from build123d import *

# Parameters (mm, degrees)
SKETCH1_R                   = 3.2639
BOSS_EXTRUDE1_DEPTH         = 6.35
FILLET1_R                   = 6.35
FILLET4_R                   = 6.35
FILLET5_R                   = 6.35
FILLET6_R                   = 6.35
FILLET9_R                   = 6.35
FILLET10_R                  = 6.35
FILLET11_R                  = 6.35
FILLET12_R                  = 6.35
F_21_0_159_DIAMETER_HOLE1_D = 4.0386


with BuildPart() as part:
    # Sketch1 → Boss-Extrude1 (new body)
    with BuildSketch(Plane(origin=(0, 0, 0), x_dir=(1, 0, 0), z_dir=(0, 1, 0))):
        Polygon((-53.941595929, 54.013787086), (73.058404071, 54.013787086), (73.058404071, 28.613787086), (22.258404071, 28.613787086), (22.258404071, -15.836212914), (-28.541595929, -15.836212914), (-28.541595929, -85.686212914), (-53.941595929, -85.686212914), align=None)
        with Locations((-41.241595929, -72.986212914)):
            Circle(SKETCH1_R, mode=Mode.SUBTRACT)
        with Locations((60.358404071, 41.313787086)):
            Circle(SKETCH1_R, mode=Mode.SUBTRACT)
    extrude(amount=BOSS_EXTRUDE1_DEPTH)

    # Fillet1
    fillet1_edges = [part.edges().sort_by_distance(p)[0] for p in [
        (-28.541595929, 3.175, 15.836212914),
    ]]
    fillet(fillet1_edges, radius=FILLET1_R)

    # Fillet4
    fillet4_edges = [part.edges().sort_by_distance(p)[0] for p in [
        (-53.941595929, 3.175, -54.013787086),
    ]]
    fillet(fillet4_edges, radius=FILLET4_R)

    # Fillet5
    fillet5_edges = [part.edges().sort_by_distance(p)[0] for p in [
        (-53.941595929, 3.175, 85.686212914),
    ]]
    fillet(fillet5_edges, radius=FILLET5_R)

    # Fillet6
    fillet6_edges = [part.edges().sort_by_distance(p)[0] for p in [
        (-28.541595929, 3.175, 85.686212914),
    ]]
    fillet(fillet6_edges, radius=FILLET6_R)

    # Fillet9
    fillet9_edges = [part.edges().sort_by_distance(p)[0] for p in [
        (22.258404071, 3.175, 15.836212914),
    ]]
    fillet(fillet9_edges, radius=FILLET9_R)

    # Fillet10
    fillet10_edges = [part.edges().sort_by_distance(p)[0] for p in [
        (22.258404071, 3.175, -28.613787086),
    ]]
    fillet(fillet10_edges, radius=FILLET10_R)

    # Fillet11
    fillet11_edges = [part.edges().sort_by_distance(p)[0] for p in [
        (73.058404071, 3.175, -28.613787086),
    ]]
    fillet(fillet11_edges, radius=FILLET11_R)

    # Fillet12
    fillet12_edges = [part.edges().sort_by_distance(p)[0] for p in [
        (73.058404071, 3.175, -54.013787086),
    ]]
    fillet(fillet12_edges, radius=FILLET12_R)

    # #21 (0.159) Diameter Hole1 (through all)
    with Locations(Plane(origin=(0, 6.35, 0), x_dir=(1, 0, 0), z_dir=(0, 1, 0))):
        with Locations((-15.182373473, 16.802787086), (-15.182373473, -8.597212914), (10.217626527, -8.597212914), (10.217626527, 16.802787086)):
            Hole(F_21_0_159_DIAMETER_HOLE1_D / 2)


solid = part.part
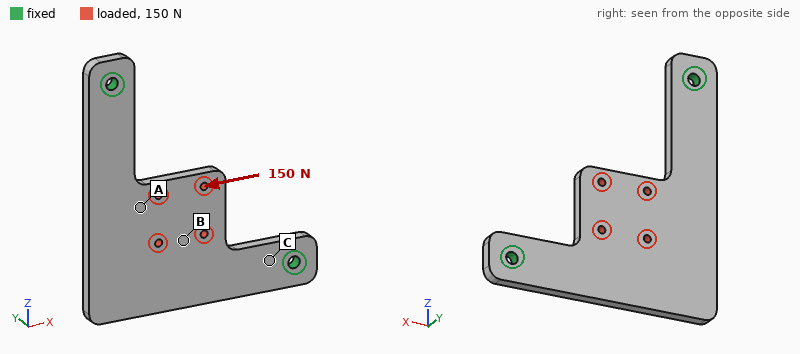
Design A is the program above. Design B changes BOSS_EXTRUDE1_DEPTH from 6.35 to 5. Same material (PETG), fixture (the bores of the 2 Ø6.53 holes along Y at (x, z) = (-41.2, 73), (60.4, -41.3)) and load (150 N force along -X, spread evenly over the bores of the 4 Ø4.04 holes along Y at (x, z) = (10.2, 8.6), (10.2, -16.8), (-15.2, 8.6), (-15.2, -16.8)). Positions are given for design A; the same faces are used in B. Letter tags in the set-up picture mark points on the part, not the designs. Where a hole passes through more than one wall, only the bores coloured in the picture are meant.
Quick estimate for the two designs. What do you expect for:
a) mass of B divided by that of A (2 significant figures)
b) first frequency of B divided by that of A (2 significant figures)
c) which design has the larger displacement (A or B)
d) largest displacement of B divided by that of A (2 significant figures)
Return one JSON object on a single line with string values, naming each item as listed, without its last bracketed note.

{"mass of B divided by that of A": "0.79", "first frequency of B divided by that of A": "0.80", "which design has the larger displacement": "B", "largest displacement of B divided by that of A": "1.3"}
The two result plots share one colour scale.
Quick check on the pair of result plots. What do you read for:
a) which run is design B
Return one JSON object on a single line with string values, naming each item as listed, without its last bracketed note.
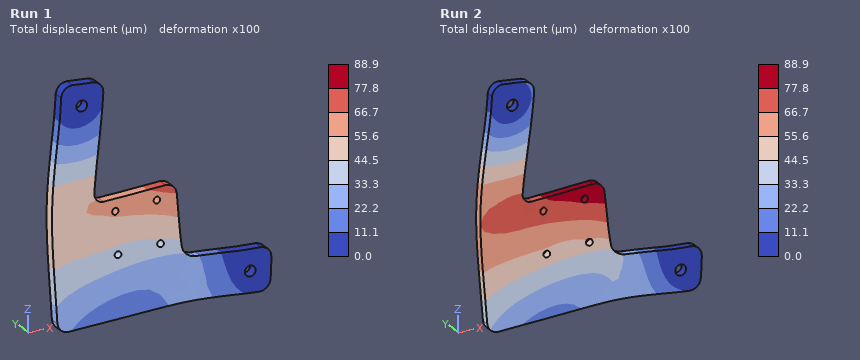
{"which run is design B": "Run 2"}
